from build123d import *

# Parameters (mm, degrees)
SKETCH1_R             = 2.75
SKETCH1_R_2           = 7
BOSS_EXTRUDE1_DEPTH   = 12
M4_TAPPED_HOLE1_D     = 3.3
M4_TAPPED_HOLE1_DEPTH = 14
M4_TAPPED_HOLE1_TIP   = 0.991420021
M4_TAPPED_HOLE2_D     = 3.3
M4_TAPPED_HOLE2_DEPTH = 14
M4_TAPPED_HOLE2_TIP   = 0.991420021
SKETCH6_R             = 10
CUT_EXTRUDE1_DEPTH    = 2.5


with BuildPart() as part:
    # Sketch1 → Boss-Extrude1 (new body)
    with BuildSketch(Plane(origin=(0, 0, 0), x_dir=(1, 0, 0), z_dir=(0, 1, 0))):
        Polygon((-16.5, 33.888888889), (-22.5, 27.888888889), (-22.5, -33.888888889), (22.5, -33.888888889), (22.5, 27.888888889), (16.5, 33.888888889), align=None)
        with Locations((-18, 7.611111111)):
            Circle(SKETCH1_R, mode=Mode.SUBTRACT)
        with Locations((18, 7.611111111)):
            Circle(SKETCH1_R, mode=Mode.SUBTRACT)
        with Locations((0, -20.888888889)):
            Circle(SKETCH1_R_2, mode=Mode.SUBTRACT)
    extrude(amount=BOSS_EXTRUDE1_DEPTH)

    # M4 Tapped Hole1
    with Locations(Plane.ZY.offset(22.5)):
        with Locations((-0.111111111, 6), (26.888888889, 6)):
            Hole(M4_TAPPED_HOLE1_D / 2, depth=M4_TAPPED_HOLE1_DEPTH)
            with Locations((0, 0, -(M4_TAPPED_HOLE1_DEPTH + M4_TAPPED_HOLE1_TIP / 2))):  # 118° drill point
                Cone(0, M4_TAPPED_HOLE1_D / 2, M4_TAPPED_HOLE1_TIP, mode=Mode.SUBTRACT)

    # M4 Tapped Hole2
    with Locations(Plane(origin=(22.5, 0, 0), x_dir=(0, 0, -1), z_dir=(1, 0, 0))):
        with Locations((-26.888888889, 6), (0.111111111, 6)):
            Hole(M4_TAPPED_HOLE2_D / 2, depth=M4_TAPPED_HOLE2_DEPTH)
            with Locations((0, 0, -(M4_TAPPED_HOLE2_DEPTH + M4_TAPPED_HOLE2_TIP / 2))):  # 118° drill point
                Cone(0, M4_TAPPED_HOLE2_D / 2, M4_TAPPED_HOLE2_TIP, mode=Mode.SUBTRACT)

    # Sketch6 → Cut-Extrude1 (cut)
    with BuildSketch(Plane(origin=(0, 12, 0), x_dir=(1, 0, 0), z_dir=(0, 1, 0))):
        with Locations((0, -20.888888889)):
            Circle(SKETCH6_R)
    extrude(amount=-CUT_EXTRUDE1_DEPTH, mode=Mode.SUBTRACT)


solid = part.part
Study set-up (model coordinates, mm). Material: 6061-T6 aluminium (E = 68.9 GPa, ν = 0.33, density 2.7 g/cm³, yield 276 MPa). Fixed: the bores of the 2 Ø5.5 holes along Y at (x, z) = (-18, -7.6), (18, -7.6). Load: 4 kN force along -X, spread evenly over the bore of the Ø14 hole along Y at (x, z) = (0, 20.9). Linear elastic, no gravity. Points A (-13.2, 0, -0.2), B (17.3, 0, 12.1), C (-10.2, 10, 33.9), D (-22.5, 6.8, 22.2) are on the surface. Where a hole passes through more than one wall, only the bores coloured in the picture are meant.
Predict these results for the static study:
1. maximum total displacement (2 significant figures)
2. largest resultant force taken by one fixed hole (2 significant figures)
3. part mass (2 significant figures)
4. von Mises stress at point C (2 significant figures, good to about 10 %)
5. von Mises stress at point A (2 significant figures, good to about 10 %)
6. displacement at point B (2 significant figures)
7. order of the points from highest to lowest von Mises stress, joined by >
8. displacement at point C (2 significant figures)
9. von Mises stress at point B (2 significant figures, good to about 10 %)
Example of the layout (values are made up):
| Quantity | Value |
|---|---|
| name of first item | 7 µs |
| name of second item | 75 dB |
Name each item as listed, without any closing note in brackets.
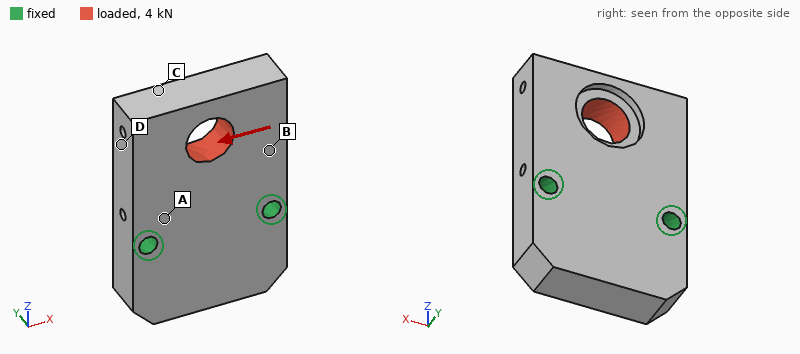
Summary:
| Quantity | Value |
|---|---|
| maximum total displacement | 28 µm |
| largest resultant force taken by one fixed hole | 3.6 kN |
| part mass | 89 g |
| von Mises stress at point C | 9.3 MPa |
| von Mises stress at point A | 20 MPa |
| displacement at point B | 11 µm |
| order of the points from highest to lowest von Mises stress, joined by > | A > B > C > D |
| displacement at point C | 25 µm |
| von Mises stress at point B | 15 MPa |
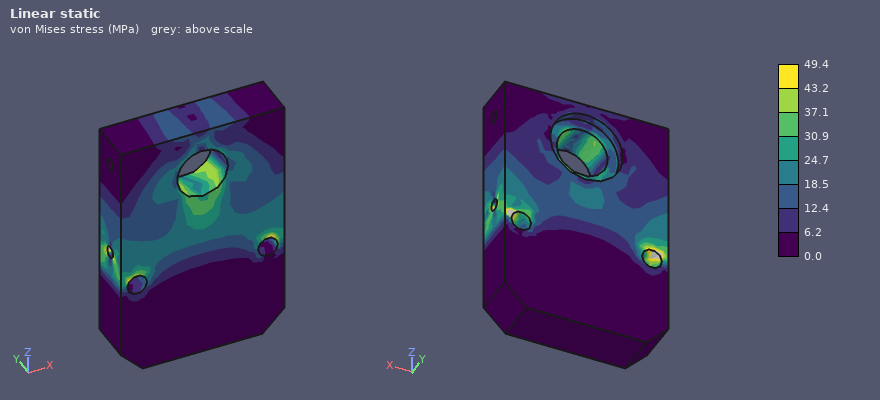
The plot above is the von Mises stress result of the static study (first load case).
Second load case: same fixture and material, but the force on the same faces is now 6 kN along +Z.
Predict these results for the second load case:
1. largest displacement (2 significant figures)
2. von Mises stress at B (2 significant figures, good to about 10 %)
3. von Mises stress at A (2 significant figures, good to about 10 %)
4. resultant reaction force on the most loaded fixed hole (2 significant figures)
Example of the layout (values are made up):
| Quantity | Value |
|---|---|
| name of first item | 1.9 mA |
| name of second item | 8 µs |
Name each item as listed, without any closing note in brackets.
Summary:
| Quantity | Value |
|---|---|
| largest displacement | 22 µm |
| von Mises stress at B | 16 MPa |
| von Mises stress at A | 22 MPa |
| resultant reaction force on the most loaded fixed hole | 3.0 kN |
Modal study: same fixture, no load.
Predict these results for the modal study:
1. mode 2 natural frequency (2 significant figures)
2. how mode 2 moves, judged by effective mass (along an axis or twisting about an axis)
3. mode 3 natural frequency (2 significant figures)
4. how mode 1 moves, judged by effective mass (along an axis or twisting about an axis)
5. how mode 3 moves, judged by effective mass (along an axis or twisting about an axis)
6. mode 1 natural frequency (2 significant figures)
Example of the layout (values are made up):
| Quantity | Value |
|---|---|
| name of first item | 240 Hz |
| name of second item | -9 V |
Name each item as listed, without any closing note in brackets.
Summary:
| Quantity | Value |
|---|---|
| mode 2 natural frequency | 9900 Hz |
| how mode 2 moves, judged by effective mass | twisting about Z |
| mode 3 natural frequency | 12 kHz |
| how mode 1 moves, judged by effective mass | along Y |
| how mode 3 moves, judged by effective mass | along Y |
| mode 1 natural frequency | 5200 Hz |
